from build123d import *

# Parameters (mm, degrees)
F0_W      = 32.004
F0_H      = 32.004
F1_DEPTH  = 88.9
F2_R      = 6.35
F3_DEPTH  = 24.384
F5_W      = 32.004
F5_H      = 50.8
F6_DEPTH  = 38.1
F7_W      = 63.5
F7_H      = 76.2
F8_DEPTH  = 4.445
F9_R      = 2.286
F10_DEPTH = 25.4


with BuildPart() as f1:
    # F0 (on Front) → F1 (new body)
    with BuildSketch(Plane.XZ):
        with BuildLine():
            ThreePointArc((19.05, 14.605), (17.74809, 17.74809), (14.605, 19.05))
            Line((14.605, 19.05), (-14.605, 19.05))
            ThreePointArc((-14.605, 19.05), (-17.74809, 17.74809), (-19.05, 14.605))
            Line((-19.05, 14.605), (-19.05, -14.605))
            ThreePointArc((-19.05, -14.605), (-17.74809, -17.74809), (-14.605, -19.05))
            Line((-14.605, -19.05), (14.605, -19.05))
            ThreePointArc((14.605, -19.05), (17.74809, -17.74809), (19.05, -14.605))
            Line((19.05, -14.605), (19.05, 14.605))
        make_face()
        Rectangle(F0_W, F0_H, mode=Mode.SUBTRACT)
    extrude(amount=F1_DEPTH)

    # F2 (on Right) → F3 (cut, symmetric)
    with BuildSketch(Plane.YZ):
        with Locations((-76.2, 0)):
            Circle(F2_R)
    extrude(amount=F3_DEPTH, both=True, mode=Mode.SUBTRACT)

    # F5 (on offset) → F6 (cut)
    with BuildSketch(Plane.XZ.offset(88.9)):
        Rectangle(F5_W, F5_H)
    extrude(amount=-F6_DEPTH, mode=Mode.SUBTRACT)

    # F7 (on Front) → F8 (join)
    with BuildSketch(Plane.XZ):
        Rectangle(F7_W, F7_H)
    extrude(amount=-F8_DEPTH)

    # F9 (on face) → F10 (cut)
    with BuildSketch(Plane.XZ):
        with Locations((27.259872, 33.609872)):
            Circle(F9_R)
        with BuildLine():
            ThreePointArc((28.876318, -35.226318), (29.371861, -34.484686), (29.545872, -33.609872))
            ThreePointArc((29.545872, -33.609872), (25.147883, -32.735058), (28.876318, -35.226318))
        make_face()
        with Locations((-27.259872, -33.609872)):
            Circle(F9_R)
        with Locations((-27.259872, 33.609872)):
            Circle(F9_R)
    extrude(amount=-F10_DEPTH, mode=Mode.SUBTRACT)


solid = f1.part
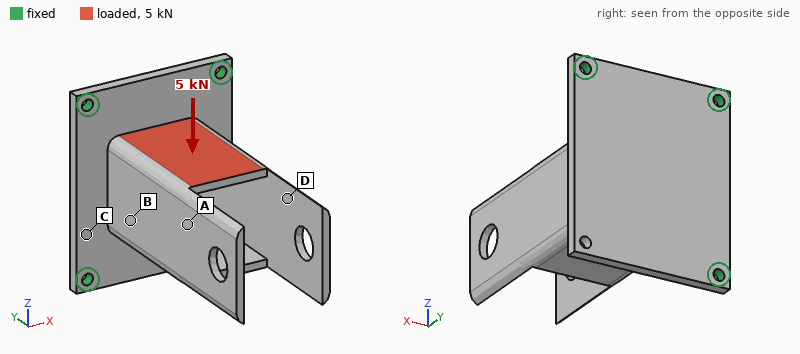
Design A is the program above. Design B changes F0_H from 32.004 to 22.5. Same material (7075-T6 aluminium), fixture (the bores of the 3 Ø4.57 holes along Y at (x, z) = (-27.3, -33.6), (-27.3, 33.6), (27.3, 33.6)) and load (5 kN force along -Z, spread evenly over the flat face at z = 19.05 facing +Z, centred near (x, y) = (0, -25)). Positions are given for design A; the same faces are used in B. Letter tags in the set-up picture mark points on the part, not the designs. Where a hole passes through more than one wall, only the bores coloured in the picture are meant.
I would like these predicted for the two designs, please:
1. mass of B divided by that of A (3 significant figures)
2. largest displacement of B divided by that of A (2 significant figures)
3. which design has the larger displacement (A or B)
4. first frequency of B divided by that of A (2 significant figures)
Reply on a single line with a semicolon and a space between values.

1.31; 0.72; A; 1.0
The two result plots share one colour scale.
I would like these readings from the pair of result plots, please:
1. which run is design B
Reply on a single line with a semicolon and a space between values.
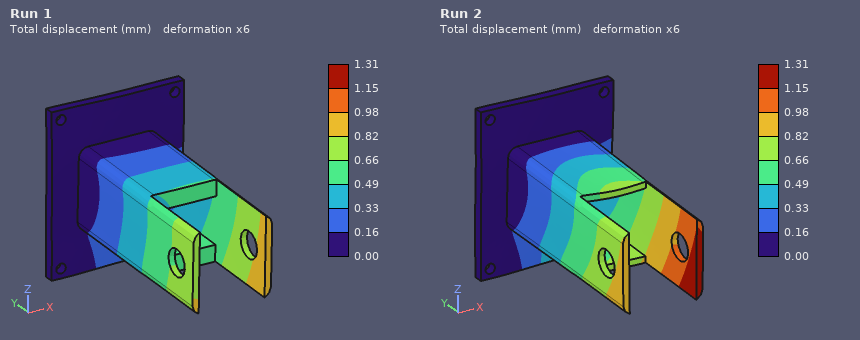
Run 1
